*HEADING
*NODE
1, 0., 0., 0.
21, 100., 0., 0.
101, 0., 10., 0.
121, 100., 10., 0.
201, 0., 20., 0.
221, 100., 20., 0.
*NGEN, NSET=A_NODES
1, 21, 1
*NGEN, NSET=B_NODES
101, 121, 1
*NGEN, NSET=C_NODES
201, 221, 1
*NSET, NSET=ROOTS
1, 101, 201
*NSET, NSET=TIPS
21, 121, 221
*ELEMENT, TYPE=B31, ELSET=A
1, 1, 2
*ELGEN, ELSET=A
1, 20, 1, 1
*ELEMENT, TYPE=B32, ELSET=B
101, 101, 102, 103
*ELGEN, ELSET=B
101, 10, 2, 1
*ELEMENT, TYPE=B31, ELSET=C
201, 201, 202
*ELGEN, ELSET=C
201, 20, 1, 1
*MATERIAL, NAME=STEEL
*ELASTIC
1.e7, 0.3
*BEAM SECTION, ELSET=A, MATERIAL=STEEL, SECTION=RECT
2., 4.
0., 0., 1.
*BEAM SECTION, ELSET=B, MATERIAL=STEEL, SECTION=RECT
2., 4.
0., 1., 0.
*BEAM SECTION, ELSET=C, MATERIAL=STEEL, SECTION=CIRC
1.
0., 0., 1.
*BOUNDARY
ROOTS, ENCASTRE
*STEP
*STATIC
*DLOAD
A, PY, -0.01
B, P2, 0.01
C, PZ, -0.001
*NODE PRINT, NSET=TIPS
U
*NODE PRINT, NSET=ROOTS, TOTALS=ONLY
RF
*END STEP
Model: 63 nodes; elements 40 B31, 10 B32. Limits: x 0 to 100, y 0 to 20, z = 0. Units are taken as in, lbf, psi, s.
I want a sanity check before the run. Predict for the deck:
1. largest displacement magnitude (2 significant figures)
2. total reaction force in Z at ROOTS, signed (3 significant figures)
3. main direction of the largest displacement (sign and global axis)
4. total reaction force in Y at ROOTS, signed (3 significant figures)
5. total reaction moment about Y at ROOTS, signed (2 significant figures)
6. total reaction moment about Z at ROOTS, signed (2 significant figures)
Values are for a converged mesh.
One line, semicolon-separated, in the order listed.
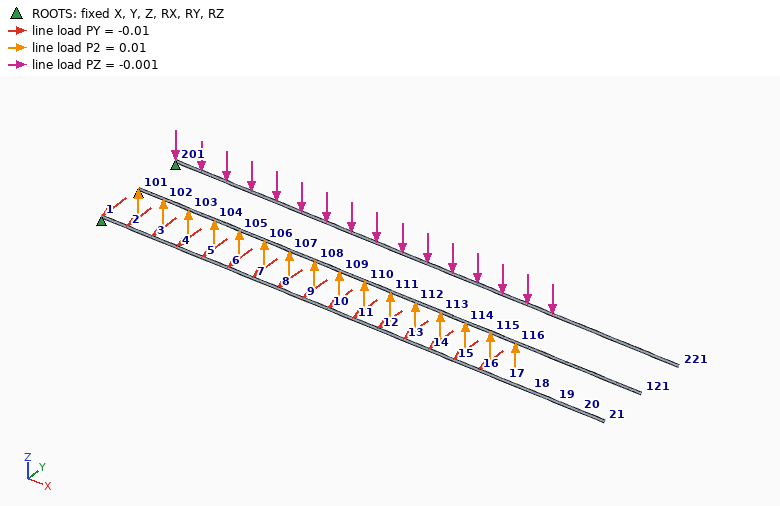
0.025 in; -0.900 lbf; -Z; 1.00 lbf; 45 lbf·in; 50 lbf·in
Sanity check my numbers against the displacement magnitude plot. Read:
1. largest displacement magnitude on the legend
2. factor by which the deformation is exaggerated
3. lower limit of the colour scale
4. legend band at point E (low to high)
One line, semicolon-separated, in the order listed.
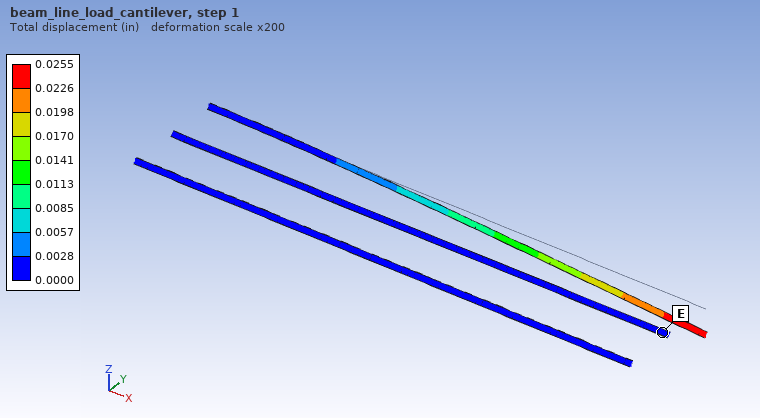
0.0255 in; 200; 0.0000 in; 0.0000 to 0.0028 in
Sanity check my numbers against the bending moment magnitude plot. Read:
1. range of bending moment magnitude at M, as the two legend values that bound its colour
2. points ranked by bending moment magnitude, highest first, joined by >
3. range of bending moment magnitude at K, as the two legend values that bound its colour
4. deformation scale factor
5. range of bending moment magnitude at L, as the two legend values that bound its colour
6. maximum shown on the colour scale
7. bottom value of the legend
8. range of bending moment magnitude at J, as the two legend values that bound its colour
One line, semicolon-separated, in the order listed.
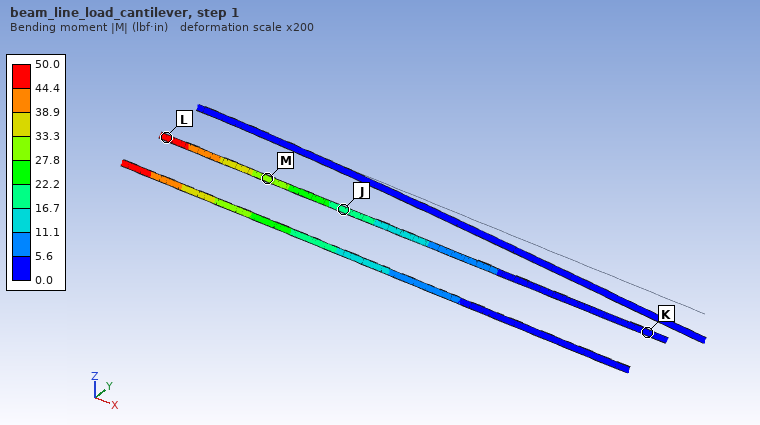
27.8 to 33.3 lbf·in; L > M > J > K; 0.0 to 5.6 lbf·in; 200; 44.4 to 50.0 lbf·in; 50.0 lbf·in; 0.0 lbf·in; 16.7 to 22.2 lbf·in
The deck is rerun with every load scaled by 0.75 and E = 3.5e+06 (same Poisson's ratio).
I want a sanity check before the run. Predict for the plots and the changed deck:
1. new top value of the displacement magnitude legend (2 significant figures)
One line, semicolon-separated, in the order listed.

0.055 in
